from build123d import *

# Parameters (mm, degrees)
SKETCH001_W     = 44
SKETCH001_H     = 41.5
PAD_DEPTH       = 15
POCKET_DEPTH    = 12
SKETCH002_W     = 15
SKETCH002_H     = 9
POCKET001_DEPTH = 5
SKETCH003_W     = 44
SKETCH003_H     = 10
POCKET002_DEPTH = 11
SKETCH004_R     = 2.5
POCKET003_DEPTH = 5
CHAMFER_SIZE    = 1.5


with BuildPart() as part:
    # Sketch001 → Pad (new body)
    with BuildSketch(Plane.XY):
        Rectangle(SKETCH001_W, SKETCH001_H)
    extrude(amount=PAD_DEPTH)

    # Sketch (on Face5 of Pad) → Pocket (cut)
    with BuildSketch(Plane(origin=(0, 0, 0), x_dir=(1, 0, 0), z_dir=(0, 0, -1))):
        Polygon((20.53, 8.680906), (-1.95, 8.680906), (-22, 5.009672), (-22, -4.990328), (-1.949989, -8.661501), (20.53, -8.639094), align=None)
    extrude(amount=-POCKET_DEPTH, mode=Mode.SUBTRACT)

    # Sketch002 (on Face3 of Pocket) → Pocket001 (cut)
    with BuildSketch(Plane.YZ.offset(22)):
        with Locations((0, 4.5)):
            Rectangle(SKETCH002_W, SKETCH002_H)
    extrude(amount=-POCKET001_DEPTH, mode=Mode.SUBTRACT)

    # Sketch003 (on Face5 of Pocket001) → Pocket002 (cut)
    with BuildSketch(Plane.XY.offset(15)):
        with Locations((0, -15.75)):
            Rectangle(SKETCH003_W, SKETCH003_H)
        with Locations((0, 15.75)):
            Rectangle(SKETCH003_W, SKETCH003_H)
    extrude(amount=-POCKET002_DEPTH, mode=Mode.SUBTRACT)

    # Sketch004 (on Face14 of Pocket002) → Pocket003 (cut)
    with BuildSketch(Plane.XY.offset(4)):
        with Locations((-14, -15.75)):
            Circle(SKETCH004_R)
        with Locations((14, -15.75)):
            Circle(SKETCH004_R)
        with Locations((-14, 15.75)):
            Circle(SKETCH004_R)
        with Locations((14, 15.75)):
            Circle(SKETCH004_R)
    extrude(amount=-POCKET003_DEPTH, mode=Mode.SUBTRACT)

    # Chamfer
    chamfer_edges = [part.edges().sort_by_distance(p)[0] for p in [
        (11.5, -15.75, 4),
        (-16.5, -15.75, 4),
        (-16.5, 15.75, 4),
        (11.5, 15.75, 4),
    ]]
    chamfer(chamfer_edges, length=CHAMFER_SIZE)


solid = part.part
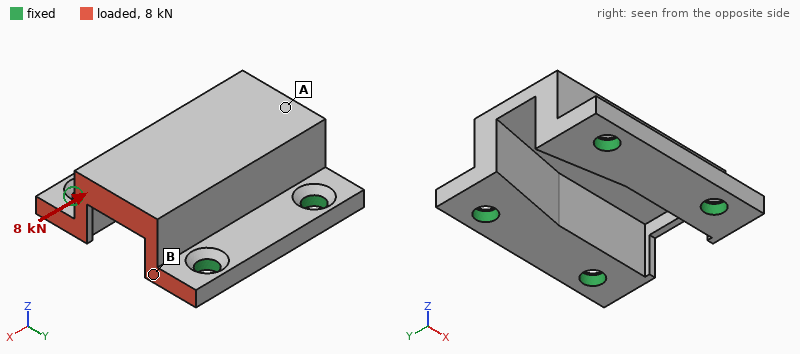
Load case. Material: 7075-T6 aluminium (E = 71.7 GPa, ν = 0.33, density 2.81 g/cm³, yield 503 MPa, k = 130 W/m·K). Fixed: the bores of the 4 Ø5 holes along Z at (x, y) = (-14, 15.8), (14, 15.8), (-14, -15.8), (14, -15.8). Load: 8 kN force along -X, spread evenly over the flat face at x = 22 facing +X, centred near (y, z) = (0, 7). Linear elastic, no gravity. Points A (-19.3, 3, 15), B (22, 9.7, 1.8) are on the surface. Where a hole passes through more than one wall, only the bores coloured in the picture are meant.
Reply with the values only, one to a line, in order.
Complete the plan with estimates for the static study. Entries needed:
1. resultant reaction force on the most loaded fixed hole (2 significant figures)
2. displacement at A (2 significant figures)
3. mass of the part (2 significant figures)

2.9 kN
24 µm
26 g
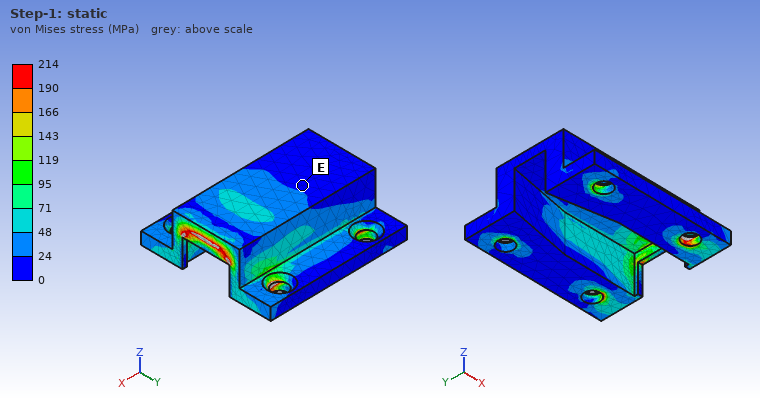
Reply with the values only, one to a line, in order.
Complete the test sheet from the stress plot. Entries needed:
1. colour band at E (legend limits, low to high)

0 to 24 MPa
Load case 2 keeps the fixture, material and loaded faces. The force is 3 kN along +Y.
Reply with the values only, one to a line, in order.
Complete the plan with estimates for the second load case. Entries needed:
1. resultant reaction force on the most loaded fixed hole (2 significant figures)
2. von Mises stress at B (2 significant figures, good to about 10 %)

1.3 kN
67 MPa
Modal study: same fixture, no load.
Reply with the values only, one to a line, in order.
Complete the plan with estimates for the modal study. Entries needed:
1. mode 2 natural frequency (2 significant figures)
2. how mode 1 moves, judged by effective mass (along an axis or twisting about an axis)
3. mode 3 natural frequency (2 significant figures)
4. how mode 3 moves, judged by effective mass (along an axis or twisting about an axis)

17 kHz
along Y
17 kHz
along X
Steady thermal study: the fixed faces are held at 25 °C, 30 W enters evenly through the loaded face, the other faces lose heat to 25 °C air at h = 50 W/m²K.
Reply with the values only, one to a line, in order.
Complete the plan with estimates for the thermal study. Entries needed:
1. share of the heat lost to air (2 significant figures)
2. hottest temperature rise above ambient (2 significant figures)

5.9 %
29 K
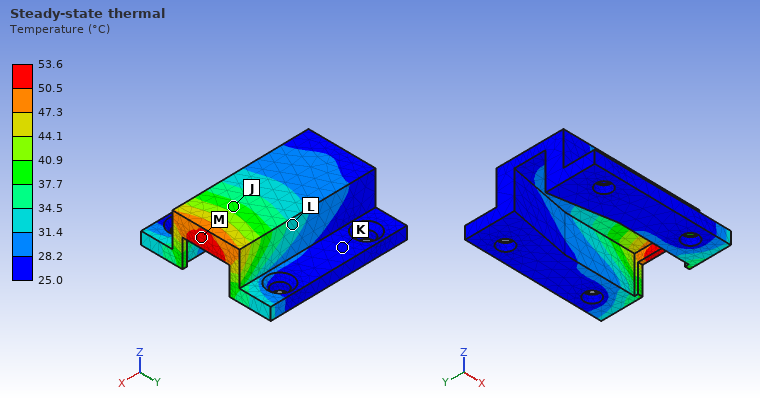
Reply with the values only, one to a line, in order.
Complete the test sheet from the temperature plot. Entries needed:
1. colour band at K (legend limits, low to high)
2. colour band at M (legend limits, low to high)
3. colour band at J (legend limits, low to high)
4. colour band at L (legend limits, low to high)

25.0 to 28.2 °C
50.5 to 53.6 °C
37.7 to 40.9 °C
31.4 to 34.5 °C
